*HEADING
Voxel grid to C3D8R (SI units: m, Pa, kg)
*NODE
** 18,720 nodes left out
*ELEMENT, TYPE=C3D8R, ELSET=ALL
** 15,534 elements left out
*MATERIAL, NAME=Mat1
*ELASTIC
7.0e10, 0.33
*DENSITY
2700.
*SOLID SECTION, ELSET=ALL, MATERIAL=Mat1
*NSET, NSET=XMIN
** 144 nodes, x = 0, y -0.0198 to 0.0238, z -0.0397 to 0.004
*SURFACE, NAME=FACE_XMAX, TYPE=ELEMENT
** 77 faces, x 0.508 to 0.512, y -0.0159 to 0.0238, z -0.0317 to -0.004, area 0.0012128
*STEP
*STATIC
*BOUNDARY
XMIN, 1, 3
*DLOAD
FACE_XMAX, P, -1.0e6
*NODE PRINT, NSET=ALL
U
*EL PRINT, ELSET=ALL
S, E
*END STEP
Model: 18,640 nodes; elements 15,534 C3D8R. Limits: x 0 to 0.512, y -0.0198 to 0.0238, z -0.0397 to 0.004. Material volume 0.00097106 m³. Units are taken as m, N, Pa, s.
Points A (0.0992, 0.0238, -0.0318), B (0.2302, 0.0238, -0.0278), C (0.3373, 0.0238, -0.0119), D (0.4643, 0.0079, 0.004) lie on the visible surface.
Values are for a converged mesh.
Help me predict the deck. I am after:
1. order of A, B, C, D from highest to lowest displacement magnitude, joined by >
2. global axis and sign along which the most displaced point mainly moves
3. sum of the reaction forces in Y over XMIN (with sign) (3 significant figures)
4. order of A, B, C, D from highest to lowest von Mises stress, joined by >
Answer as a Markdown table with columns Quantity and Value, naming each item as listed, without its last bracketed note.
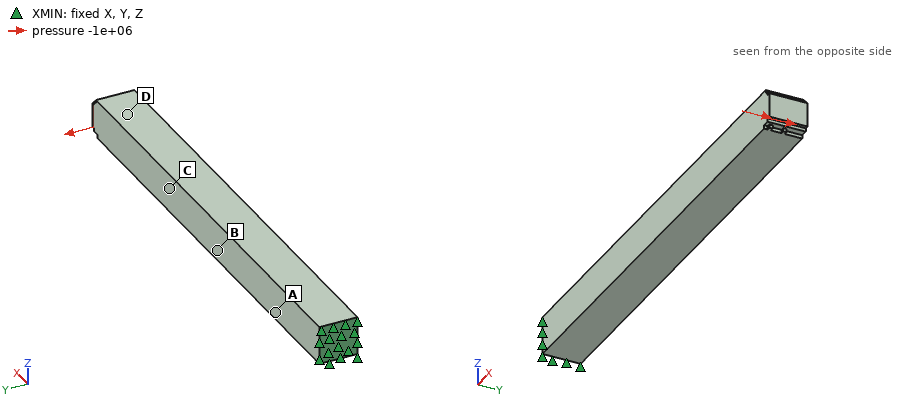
| Quantity | Value |
|---|---|
| order of A, B, C, D from highest to lowest displacement magnitude, joined by > | D > C > B > A |
| global axis and sign along which the most displaced point mainly moves | +Y |
| sum of the reaction forces in Y over XMIN (with sign) | -1210 N |
| order of A, B, C, D from highest to lowest von Mises stress, joined by > | A > B > C > D |
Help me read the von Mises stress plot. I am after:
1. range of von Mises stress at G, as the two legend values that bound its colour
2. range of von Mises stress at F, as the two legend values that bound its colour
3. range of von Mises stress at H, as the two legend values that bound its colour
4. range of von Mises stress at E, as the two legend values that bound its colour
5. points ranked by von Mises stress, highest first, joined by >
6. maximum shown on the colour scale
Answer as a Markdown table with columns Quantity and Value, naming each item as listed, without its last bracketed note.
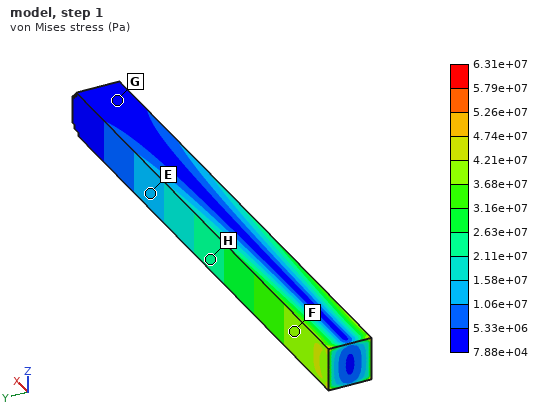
| Quantity | Value |
|---|---|
| range of von Mises stress at G, as the two legend values that bound its colour | 7.88e+04 to 5.33e+06 Pa |
| range of von Mises stress at F, as the two legend values that bound its colour | 3.68e+07 to 4.21e+07 Pa |
| range of von Mises stress at H, as the two legend values that bound its colour | 2.11e+07 to 2.63e+07 Pa |
| range of von Mises stress at E, as the two legend values that bound its colour | 1.06e+07 to 1.58e+07 Pa |
| points ranked by von Mises stress, highest first, joined by > | F > H > E > G |
| maximum shown on the colour scale | 6.31e+07 Pa |
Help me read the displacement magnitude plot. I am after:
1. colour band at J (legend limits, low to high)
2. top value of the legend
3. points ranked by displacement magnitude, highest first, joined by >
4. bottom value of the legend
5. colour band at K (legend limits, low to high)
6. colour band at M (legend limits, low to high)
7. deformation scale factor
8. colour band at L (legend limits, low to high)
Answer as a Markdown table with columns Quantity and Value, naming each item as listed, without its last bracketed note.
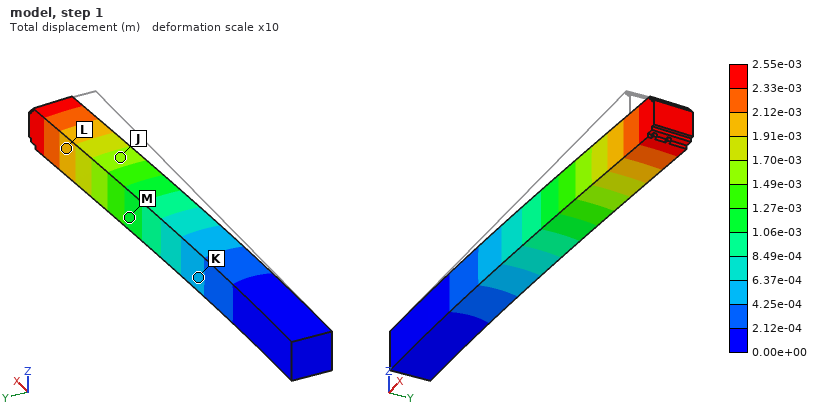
| Quantity | Value |
|---|---|
| colour band at J | 1.49e-03 to 1.70e-03 m |
| top value of the legend | 2.55e-03 m |
| points ranked by displacement magnitude, highest first, joined by > | L > J > M > K |
| bottom value of the legend | 0.00e+00 m |
| colour band at K | 4.25e-04 to 6.37e-04 m |
| colour band at M | 1.06e-03 to 1.27e-03 m |
| deformation scale factor | 10 |
| colour band at L | 1.91e-03 to 2.12e-03 m |
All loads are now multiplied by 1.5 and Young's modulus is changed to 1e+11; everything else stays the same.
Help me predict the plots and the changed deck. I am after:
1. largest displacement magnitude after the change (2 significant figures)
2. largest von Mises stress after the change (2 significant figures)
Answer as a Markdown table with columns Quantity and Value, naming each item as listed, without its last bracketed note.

| Quantity | Value |
|---|---|
| largest displacement magnitude after the change | 0.0027 m |
| largest von Mises stress after the change | 9.5e+07 Pa |
